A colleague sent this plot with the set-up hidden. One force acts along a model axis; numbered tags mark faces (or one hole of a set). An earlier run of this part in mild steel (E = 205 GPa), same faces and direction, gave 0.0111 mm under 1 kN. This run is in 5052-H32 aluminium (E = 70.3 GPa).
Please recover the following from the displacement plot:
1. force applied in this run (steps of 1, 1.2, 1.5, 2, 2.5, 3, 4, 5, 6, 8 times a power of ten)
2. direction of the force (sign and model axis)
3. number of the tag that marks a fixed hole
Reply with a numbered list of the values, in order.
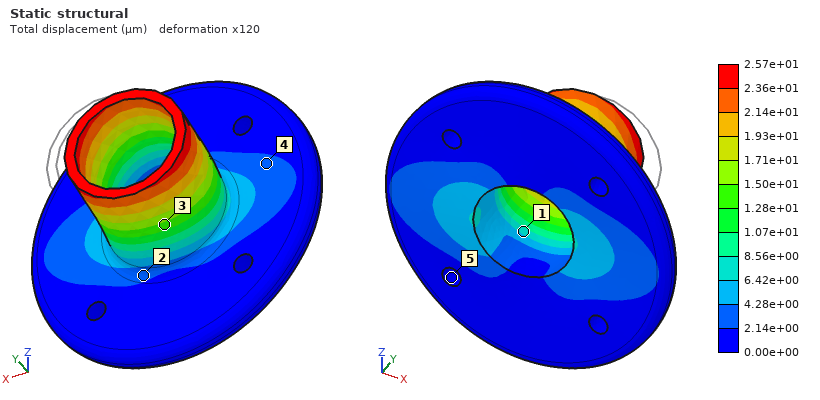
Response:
1. 800 N
2. -X
3. 5
